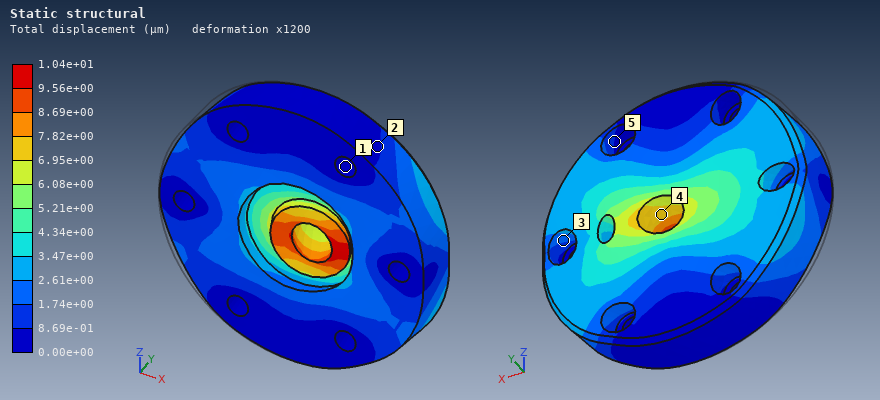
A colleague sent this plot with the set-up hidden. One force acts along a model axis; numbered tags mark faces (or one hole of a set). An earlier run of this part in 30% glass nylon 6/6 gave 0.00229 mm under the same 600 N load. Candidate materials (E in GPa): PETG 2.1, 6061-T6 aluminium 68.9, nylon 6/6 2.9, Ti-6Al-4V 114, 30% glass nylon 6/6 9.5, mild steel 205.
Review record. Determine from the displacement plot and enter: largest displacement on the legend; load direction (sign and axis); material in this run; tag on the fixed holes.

1.04e+01 µm
+X
PETG
1
